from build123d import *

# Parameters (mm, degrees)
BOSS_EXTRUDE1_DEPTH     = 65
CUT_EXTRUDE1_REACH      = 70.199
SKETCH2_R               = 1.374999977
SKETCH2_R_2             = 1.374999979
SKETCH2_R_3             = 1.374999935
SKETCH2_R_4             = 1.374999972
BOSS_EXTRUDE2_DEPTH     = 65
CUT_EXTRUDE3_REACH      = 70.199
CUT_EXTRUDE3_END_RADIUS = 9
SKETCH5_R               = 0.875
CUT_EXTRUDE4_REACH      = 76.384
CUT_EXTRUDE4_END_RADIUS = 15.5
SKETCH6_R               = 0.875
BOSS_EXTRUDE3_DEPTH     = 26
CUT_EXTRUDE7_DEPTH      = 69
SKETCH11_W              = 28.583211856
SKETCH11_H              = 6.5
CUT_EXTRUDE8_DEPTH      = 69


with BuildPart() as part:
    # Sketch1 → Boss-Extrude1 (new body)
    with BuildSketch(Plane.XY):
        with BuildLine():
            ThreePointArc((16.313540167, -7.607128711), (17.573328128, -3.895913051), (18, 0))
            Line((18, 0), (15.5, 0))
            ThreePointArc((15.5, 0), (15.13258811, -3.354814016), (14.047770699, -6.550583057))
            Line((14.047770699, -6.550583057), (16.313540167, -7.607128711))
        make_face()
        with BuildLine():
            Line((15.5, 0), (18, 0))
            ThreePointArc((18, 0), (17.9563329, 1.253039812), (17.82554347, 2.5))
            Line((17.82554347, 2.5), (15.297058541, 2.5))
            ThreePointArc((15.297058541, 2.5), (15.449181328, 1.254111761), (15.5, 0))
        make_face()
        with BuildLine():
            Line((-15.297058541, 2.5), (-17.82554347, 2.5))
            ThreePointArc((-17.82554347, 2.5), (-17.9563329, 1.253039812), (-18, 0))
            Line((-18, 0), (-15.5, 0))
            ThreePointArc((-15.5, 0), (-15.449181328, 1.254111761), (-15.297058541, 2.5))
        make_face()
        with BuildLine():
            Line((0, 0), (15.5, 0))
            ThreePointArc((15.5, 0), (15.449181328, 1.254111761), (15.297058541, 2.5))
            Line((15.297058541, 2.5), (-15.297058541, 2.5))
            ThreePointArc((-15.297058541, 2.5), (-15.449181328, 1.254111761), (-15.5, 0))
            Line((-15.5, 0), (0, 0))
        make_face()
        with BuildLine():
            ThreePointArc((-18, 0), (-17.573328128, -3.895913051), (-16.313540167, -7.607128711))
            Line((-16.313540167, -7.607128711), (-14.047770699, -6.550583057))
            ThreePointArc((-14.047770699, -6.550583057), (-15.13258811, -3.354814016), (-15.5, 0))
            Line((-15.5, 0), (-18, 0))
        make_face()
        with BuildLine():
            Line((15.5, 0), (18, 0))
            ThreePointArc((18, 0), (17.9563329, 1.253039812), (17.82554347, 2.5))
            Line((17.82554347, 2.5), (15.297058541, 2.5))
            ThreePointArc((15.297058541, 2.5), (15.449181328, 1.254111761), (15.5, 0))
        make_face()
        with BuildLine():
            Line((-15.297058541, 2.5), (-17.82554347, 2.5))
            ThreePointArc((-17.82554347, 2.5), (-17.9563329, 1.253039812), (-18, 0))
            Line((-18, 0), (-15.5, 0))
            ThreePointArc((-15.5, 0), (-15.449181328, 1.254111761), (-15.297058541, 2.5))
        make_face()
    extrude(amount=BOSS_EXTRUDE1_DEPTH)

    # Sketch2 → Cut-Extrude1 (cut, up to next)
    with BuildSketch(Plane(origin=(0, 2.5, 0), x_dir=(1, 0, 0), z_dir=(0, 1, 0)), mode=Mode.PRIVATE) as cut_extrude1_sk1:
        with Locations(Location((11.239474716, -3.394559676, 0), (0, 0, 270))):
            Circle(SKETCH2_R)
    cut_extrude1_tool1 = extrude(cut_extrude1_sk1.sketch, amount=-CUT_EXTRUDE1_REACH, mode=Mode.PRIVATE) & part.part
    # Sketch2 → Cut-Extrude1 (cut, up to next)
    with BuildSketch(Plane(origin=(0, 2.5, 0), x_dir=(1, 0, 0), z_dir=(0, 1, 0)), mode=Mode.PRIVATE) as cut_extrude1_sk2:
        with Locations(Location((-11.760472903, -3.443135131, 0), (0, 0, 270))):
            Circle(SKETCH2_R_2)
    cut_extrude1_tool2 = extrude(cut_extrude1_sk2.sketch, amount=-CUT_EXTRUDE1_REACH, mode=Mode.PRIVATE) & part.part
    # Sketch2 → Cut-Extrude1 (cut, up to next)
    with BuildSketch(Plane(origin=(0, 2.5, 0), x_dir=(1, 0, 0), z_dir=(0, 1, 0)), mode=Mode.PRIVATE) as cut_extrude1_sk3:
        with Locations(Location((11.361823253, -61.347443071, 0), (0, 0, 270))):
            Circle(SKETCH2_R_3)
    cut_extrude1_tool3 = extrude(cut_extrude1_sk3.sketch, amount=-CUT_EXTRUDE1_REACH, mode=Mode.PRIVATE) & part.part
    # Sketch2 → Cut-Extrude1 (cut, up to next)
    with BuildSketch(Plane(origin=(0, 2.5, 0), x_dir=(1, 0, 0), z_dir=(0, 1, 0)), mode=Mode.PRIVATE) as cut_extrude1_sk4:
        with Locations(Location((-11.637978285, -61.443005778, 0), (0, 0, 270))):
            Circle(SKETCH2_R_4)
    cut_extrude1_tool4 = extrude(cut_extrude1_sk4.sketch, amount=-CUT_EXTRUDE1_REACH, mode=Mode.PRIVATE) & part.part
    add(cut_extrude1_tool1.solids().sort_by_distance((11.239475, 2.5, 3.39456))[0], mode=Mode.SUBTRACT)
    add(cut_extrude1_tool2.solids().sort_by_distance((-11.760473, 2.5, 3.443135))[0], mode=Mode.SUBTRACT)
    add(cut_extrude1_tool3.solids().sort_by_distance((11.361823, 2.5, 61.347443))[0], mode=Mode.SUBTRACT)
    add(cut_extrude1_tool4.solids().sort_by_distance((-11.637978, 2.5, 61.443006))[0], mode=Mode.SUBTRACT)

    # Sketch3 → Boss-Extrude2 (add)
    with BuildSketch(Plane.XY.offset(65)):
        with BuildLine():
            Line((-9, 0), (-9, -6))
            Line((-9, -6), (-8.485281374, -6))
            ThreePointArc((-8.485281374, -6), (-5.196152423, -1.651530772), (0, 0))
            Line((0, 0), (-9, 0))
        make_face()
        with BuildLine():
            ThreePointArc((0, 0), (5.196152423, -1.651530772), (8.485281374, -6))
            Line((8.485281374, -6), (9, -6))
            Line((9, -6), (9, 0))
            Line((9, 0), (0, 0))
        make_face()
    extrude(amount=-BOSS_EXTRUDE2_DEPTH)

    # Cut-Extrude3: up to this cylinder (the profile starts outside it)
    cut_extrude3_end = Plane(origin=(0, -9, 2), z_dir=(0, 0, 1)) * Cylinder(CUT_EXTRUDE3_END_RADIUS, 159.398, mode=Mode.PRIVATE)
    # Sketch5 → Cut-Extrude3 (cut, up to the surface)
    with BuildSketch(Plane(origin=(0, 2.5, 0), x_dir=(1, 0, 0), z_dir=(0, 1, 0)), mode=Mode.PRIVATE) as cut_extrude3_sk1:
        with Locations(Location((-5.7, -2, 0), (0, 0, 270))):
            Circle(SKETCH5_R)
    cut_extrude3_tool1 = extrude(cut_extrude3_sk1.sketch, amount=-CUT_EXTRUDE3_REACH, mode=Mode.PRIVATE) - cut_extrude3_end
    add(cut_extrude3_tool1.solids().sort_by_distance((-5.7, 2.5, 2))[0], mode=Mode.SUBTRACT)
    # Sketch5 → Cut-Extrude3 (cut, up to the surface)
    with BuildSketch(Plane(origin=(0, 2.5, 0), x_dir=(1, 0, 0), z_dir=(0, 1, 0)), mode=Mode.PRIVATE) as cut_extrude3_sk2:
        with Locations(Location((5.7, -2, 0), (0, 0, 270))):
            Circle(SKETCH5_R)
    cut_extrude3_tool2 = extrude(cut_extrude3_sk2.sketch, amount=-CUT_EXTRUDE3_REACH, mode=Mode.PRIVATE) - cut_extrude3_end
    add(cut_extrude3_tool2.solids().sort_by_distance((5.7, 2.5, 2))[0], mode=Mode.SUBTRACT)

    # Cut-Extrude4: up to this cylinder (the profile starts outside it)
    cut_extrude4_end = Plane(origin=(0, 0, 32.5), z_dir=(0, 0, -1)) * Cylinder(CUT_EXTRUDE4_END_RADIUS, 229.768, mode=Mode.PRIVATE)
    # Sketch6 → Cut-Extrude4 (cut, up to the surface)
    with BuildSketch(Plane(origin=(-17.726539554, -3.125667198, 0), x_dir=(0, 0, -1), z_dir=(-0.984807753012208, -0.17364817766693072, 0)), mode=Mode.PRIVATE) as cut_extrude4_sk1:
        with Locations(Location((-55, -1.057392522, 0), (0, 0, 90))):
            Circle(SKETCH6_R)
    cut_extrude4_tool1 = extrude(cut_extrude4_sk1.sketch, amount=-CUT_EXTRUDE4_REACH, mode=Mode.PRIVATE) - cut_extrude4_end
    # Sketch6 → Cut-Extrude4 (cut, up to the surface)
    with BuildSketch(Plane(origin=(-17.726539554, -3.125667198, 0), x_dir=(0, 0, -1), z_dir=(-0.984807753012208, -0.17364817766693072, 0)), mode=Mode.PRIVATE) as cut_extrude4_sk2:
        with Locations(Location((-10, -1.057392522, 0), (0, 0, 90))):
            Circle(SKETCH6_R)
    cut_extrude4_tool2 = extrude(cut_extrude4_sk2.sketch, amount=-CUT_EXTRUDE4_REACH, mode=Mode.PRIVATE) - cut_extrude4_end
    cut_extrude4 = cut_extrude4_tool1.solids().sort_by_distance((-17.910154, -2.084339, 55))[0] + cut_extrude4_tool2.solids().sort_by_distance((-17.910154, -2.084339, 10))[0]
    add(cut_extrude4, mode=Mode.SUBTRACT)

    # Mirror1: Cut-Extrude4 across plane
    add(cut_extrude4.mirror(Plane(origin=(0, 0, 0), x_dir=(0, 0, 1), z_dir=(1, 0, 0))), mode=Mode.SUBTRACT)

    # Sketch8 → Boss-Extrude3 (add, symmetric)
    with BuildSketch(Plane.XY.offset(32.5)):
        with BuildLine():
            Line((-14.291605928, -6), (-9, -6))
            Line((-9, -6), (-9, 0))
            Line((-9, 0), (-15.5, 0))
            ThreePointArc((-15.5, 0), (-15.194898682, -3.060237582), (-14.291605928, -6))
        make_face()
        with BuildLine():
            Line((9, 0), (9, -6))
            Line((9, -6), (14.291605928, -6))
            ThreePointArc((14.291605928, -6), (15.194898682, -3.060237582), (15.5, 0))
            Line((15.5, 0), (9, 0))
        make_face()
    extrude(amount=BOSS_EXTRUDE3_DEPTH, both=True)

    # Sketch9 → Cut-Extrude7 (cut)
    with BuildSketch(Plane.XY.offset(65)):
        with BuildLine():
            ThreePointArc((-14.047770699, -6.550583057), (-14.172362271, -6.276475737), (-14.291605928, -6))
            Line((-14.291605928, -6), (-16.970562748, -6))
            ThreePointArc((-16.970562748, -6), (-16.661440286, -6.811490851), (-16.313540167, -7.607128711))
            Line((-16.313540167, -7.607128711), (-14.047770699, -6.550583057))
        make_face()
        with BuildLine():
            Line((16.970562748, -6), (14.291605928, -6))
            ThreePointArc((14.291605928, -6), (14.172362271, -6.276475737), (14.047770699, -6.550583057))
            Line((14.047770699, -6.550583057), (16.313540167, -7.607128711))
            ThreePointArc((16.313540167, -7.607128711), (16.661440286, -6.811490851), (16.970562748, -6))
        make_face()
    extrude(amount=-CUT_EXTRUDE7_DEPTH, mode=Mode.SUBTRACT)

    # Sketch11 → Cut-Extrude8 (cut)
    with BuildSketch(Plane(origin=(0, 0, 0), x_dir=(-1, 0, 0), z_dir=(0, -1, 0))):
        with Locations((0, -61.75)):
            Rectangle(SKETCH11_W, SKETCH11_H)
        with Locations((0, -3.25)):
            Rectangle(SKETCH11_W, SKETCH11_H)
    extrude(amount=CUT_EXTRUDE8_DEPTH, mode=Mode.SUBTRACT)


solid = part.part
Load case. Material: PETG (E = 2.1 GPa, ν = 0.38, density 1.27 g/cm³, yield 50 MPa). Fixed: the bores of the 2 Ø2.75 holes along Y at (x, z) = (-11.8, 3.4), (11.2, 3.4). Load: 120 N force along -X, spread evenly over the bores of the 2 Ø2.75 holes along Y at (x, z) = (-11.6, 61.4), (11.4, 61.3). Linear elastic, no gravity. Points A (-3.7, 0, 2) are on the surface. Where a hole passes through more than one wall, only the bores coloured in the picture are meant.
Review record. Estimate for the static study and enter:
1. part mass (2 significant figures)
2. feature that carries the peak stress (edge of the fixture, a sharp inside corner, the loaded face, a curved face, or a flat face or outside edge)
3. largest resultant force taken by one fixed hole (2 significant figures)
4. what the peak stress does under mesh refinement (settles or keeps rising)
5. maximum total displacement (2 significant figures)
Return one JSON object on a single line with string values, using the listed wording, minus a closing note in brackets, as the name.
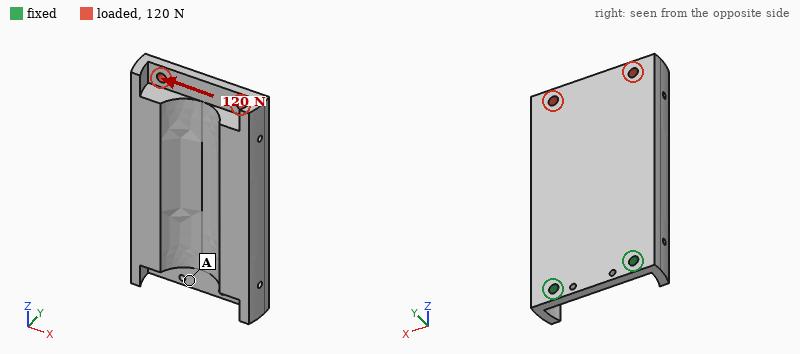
{"part mass": "17 g", "feature that carries the peak stress": "edge of the fixture", "largest resultant force taken by one fixed hole": "290 N", "what the peak stress does under mesh refinement": "keeps rising", "maximum total displacement": "0.53 mm"}
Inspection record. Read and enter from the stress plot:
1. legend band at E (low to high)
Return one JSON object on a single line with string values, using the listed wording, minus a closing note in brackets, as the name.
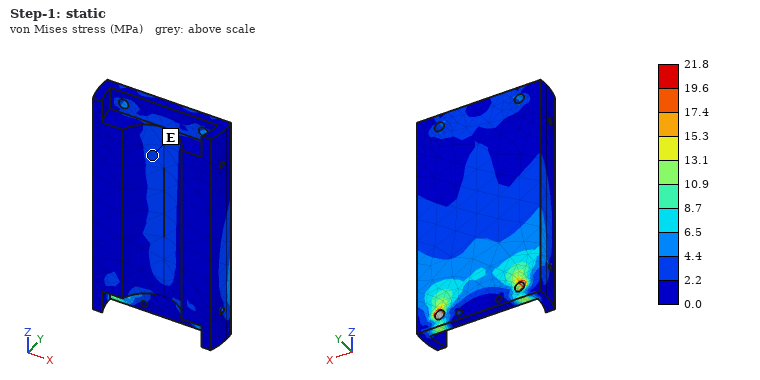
{"legend band at E": "2.2 to 4.4 MPa"}
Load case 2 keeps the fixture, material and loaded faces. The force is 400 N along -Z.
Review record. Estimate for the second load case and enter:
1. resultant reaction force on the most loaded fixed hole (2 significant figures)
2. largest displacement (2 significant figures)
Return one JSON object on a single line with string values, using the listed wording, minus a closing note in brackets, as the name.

{"resultant reaction force on the most loaded fixed hole": "200 N", "largest displacement": "0.64 mm"}
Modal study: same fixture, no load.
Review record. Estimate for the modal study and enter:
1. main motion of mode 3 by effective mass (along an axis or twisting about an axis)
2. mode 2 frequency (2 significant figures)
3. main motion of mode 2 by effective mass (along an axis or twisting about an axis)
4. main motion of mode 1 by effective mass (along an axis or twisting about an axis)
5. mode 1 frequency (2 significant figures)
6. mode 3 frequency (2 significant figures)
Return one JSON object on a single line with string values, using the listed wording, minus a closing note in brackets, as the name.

{"main motion of mode 3 by effective mass": "along X", "mode 2 frequency": "850 Hz", "main motion of mode 2 by effective mass": "twisting about Z", "main motion of mode 1 by effective mass": "along Y", "mode 1 frequency": "190 Hz", "mode 3 frequency": "1100 Hz"}
